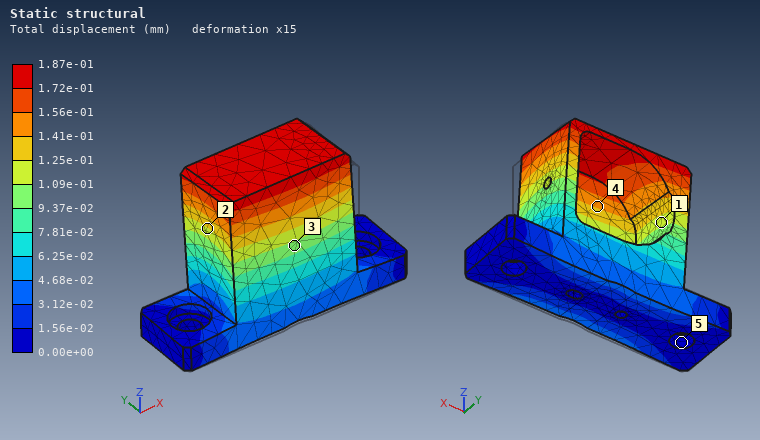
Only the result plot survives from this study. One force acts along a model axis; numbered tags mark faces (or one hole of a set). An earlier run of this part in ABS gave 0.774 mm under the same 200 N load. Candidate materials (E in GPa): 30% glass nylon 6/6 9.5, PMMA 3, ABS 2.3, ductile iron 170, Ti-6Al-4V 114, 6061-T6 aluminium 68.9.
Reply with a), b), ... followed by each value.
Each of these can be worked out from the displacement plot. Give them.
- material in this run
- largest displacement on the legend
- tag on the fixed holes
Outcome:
a) 30% glass nylon 6/6
b) 1.87e-01 mm
c) 5
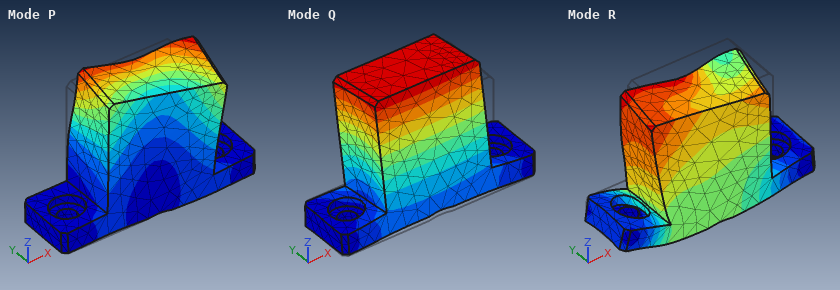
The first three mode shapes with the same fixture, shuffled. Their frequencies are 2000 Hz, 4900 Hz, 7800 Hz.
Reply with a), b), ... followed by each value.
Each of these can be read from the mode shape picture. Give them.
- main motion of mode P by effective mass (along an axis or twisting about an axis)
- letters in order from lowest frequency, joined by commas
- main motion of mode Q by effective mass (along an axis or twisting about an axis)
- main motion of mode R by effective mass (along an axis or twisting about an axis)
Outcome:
a) along X
b) Q, P, R
c) along Y
d) along Z
